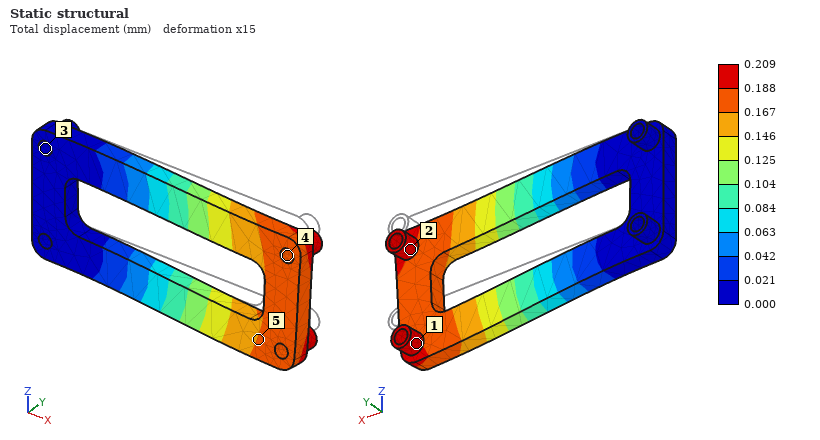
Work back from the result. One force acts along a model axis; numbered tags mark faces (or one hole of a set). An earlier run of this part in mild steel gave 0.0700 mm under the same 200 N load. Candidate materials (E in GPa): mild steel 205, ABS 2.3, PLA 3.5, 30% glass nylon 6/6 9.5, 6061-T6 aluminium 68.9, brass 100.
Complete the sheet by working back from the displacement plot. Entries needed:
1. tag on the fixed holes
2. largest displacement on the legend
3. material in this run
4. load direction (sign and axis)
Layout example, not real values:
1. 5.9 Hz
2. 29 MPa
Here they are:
1. 3
2. 0.209 mm
3. 6061-T6 aluminium
4. -Z
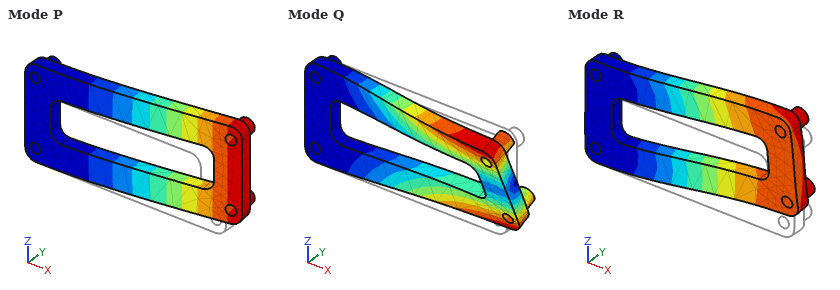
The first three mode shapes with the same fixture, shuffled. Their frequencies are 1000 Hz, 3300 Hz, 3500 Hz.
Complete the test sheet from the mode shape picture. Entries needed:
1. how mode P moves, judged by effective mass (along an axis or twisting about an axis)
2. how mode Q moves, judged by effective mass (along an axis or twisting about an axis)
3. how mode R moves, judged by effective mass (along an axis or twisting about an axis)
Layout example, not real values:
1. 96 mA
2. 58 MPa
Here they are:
1. along Y
2. twisting about X
3. along Z
